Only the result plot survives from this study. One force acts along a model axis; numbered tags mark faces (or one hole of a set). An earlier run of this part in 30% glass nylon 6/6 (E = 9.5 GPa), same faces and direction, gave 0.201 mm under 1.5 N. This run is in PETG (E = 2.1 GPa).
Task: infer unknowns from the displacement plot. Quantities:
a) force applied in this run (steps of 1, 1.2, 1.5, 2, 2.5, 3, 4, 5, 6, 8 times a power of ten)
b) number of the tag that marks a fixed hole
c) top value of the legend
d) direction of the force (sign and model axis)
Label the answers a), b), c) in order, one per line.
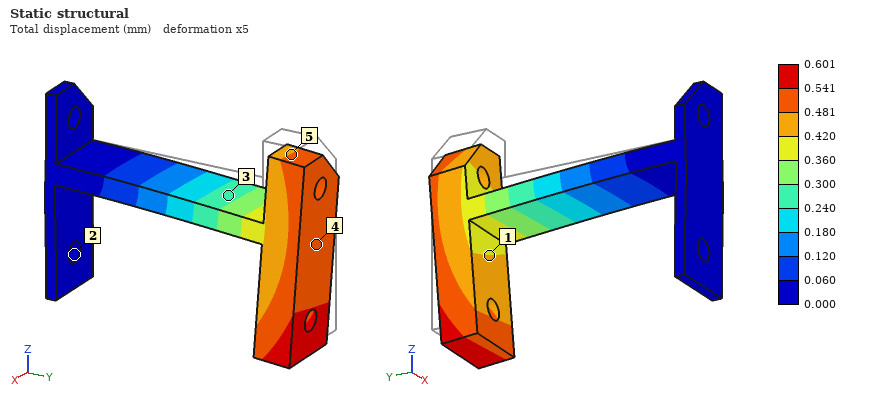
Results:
a) 1 N
b) 2
c) 0.601 mm
d) -Z
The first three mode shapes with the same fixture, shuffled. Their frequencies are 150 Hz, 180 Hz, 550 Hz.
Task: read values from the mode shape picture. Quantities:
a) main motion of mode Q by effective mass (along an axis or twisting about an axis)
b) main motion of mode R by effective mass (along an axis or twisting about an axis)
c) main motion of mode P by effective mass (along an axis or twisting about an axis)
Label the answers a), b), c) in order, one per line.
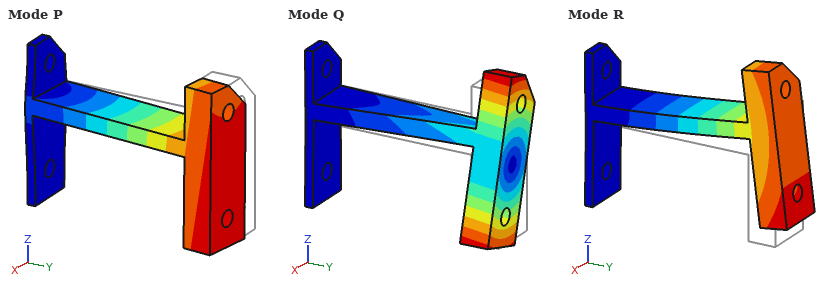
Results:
a) twisting about Y
b) along Z
c) along X
